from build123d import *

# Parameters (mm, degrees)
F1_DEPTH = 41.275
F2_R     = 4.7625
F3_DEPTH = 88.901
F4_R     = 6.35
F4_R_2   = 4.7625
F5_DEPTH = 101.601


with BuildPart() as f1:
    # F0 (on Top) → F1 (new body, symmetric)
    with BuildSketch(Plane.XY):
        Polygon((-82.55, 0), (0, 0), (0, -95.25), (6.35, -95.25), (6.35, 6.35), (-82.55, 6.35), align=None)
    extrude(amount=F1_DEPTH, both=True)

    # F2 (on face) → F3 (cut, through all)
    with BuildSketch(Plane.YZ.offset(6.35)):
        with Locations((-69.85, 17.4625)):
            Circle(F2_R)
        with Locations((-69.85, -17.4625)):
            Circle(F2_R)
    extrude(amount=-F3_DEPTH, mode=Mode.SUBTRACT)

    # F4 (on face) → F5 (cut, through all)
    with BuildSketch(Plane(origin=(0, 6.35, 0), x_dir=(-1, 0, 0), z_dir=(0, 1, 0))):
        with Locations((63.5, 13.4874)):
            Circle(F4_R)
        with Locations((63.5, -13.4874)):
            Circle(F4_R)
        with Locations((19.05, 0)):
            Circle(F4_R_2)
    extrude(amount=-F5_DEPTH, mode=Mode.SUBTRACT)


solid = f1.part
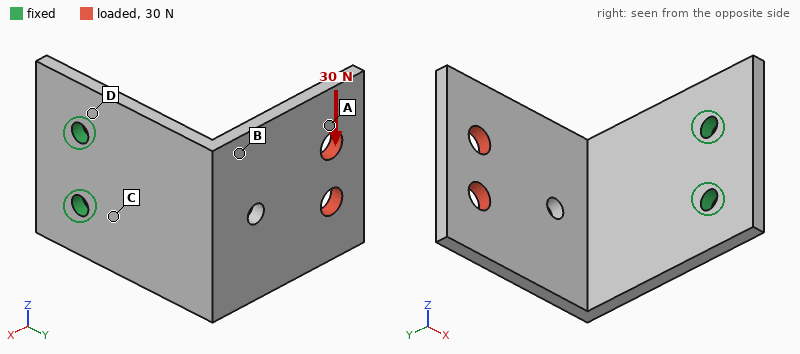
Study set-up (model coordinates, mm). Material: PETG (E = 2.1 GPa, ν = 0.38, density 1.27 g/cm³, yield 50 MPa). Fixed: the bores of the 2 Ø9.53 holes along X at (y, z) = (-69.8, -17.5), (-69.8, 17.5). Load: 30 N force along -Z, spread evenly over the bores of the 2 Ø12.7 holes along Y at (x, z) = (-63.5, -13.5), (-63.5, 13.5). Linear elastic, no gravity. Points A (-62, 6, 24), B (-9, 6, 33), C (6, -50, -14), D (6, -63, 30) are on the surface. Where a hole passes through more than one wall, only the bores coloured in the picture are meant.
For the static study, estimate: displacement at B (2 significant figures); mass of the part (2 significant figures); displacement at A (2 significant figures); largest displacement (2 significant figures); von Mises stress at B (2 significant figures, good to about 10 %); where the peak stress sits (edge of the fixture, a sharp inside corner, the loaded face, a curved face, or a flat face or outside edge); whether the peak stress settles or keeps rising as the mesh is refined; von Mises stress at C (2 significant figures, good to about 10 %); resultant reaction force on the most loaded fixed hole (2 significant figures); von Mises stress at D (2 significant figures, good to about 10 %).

0.64 mm
120 g
1.2 mm
1.7 mm
1.2 MPa
edge of the fixture
keeps rising
2.1 MPa
67 N
2.5 MPa
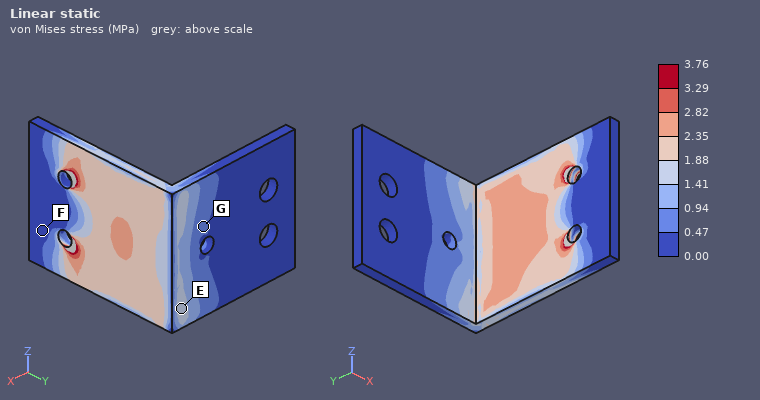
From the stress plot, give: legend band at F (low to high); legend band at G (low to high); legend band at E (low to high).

0.00 to 0.47 MPa
0.47 to 0.94 MPa
1.41 to 1.88 MPa
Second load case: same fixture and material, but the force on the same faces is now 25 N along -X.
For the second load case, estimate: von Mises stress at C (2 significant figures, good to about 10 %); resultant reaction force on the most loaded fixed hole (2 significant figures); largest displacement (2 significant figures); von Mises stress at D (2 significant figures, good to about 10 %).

2.2 MPa
13 N
1.6 mm
2.0 MPa
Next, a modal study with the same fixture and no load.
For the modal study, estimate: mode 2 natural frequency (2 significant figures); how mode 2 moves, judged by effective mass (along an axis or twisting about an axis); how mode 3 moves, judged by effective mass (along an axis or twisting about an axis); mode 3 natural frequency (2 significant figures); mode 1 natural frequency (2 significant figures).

130 Hz
along Z
along X
210 Hz
76 Hz
